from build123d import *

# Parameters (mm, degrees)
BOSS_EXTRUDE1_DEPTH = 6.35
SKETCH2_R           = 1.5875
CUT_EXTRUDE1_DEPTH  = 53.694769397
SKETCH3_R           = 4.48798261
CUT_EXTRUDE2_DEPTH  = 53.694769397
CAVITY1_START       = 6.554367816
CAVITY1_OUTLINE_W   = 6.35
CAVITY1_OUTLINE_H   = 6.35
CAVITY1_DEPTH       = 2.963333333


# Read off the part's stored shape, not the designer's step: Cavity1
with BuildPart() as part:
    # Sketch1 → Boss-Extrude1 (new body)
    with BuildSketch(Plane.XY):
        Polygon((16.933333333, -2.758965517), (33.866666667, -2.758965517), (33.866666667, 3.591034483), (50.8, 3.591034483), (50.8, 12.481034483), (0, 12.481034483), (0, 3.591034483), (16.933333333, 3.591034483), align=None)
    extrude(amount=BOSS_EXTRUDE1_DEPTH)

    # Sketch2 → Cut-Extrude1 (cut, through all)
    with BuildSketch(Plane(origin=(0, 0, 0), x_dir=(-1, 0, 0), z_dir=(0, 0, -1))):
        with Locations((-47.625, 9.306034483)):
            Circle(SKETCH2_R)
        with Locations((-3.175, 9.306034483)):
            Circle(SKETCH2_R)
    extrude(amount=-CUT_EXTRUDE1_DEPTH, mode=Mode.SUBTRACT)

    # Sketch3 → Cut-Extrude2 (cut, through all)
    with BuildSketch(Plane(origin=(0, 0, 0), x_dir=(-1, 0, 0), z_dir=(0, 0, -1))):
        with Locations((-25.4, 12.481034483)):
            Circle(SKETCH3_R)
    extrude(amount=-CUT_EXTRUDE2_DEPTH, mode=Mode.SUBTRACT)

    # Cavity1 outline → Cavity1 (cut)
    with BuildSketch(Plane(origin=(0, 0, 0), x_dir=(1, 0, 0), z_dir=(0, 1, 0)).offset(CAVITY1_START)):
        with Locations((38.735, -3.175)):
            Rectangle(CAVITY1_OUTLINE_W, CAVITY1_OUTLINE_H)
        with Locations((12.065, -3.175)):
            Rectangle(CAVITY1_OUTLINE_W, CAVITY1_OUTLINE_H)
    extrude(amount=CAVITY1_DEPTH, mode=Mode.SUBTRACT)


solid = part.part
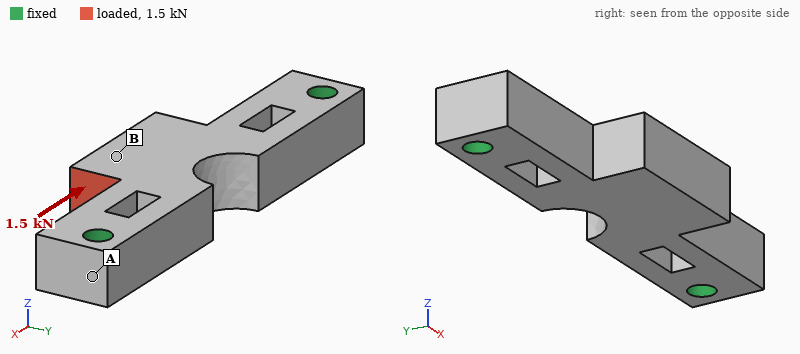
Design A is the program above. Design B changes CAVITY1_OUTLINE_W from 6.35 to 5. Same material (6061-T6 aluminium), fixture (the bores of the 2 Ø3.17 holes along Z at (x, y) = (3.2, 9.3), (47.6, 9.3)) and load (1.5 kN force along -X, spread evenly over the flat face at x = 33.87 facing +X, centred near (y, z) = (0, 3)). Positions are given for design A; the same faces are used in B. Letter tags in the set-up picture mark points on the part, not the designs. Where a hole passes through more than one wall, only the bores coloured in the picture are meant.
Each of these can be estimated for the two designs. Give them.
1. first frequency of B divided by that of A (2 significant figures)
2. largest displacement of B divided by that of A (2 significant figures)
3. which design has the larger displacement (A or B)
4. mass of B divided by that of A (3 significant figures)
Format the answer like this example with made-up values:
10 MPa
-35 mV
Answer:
1.0
0.90
A
1.02
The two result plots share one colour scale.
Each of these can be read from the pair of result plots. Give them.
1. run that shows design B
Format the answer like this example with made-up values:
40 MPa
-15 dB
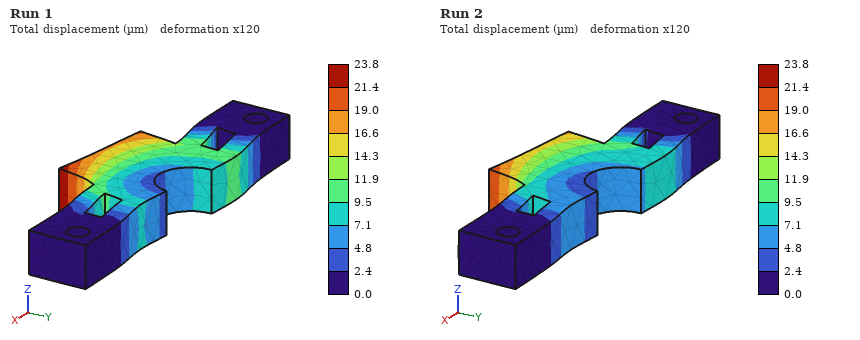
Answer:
Run 2
